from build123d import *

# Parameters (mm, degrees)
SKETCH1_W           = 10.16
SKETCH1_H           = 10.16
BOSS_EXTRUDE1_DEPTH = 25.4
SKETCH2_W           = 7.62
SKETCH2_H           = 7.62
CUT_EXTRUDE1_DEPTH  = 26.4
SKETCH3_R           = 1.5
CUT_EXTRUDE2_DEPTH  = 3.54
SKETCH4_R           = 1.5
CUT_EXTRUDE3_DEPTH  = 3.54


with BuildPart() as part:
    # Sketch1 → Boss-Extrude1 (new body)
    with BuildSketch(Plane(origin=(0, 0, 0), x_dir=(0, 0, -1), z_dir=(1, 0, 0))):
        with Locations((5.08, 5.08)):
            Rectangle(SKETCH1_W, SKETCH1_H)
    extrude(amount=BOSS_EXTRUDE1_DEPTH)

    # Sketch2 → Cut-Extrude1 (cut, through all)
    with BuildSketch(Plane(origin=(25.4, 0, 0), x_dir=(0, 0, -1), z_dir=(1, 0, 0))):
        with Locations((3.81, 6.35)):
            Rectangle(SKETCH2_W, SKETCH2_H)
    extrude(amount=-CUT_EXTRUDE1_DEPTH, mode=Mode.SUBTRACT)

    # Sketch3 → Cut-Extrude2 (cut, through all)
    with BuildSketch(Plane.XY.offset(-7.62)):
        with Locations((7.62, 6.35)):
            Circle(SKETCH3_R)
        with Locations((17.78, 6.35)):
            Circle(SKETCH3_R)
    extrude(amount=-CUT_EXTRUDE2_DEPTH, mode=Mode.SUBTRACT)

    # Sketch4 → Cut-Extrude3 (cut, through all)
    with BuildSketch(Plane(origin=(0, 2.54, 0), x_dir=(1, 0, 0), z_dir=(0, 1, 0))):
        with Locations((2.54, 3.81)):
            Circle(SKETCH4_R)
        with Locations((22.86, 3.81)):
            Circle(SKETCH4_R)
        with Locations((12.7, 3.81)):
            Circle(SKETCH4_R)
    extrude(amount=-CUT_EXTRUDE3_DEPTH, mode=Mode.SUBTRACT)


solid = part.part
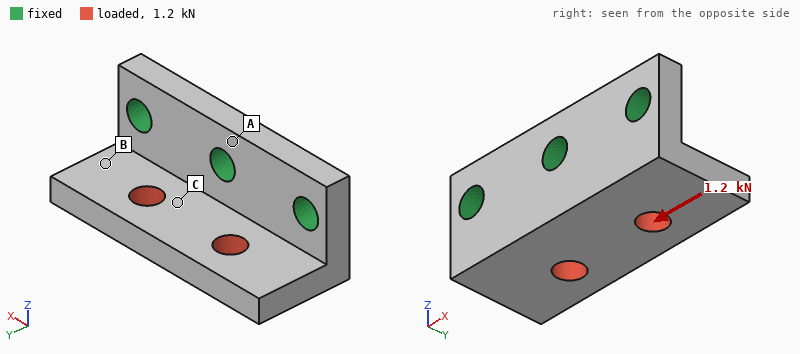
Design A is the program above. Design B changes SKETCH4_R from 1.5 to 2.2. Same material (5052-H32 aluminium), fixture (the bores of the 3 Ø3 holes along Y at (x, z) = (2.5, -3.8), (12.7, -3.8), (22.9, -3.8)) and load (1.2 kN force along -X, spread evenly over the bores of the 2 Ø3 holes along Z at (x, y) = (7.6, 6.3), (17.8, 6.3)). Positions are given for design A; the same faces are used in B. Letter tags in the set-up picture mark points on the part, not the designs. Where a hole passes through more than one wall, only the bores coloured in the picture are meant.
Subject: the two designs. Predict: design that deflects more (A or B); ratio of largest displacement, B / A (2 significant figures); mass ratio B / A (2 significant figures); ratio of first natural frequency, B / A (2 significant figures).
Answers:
A
0.73
0.94
1.1
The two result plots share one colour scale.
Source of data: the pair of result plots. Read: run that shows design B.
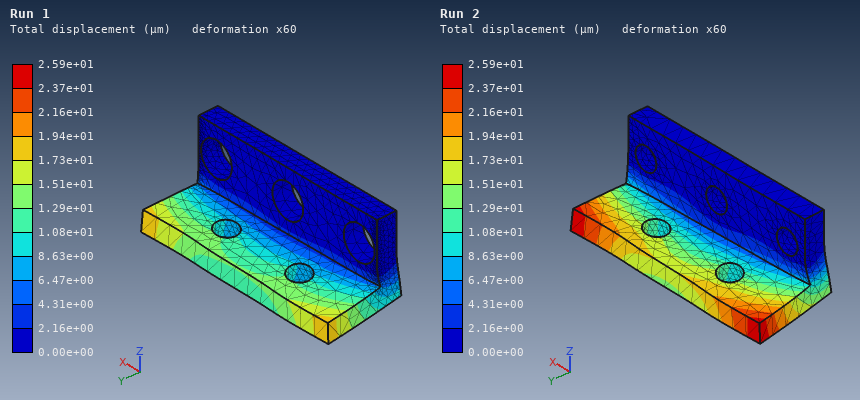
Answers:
Run 1
